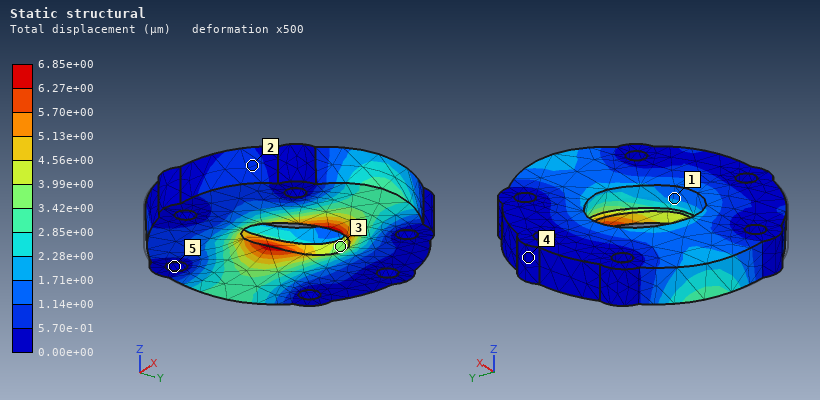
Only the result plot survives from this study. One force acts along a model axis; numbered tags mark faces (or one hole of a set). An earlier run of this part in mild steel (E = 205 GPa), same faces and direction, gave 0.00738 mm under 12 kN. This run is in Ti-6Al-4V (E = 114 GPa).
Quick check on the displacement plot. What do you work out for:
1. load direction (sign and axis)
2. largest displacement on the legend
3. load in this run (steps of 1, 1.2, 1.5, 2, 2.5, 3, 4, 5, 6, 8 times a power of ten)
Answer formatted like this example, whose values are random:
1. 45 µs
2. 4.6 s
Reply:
1. +X
2. 6.85e+00 µm
3. 6 kN
